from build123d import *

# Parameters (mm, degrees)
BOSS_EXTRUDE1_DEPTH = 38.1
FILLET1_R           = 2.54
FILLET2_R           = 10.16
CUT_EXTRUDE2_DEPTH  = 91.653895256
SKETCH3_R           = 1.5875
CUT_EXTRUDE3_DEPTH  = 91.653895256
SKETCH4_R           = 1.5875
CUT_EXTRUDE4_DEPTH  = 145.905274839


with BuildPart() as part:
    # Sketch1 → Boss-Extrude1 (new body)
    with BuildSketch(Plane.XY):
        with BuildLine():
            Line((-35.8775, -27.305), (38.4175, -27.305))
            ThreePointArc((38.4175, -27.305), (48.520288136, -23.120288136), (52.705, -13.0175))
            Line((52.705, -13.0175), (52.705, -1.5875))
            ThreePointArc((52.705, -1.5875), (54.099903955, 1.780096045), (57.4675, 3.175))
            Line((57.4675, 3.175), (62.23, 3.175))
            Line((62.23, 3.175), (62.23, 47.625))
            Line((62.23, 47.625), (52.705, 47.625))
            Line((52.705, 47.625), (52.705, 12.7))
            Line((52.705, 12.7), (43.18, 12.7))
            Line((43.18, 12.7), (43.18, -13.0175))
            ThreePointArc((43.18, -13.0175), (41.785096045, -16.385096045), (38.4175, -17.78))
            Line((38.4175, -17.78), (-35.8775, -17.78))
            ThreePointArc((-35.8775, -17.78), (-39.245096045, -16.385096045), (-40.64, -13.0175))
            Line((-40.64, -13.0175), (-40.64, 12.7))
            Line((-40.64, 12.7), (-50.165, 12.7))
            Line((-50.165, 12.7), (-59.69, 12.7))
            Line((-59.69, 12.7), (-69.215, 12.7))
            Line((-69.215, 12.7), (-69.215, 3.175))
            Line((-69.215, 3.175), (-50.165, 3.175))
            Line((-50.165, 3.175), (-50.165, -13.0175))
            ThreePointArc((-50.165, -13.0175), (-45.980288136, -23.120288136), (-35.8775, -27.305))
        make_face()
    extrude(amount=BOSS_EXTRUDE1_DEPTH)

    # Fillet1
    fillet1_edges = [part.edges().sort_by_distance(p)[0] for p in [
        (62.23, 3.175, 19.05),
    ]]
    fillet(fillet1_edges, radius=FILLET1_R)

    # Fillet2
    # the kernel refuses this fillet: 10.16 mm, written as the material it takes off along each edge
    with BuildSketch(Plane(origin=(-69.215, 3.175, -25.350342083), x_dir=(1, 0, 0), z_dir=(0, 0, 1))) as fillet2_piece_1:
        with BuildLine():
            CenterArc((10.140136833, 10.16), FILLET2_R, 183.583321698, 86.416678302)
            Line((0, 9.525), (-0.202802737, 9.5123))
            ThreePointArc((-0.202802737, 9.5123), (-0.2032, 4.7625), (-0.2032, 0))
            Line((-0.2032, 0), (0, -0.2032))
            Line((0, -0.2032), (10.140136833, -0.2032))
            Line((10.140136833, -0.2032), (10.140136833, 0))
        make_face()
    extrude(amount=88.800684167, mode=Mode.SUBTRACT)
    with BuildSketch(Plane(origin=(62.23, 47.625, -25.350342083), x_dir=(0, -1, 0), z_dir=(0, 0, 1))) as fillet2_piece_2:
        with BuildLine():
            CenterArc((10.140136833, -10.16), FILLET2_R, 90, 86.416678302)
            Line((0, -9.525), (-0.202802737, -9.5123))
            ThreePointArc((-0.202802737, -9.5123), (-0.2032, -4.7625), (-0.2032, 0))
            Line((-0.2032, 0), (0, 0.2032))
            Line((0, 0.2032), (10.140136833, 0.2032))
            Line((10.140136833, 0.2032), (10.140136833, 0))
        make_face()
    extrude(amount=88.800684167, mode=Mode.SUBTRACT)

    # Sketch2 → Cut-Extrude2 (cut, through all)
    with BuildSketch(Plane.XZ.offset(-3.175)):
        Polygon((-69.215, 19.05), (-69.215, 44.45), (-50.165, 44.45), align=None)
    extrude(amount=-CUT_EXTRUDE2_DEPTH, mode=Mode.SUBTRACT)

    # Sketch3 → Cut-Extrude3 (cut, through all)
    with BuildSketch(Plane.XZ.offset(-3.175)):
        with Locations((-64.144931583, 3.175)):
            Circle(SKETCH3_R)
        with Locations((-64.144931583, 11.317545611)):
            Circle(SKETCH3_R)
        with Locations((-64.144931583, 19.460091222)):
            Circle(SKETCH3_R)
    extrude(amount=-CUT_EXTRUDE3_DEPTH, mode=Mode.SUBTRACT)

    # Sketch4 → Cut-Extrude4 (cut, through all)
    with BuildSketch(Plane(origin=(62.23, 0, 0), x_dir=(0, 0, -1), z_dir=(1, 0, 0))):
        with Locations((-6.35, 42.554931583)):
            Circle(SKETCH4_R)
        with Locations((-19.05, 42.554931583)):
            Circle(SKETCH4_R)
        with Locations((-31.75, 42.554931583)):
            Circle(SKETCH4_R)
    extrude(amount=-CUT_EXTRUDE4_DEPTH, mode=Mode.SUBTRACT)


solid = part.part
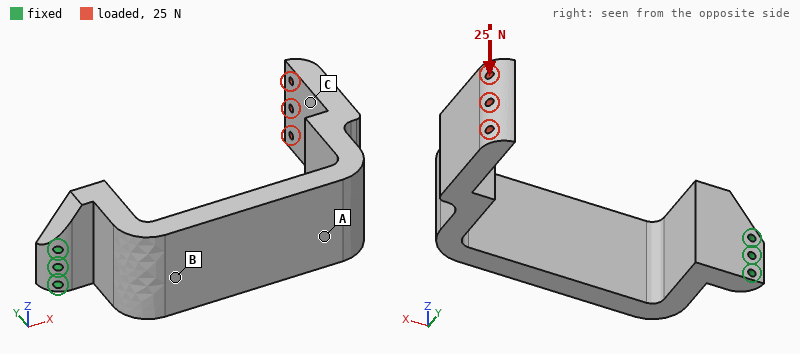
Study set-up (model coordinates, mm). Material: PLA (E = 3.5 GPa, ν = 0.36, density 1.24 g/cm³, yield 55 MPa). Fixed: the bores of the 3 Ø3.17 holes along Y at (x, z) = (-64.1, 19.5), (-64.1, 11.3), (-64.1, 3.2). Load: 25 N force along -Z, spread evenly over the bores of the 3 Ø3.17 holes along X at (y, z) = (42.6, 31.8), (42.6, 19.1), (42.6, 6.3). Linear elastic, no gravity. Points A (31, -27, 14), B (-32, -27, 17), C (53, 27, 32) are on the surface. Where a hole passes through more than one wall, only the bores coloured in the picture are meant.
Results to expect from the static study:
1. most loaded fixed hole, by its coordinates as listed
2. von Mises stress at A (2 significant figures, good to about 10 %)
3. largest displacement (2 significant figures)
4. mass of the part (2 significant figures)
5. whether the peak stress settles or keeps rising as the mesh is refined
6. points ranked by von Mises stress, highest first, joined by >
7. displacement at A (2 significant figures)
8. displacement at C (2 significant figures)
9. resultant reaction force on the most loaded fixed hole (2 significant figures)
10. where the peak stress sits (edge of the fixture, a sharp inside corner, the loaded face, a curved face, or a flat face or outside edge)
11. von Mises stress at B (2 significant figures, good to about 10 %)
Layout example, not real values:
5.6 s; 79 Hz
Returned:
(-64.1, 19.5); 2.4 MPa; 1.7 mm; 95 g; keeps rising; B > A > C; 0.41 mm; 1.4 mm; 180 N; edge of the fixture; 3.2 MPa
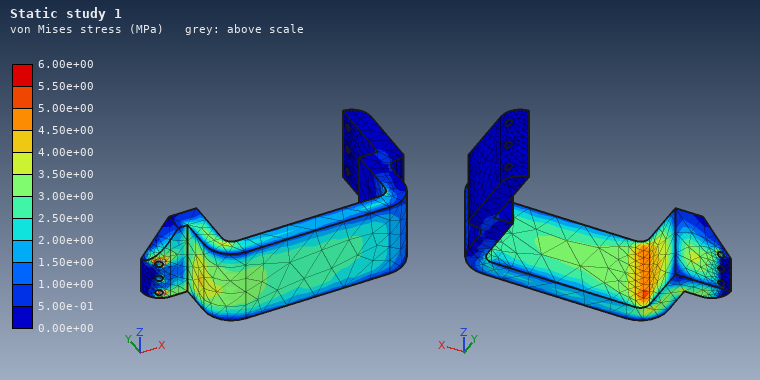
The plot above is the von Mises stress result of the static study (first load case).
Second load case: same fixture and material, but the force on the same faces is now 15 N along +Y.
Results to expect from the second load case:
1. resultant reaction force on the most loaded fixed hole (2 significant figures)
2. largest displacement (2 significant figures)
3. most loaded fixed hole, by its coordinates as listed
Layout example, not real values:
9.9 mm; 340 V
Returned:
20 N; 1.7 mm; (-64.1, 11.3)
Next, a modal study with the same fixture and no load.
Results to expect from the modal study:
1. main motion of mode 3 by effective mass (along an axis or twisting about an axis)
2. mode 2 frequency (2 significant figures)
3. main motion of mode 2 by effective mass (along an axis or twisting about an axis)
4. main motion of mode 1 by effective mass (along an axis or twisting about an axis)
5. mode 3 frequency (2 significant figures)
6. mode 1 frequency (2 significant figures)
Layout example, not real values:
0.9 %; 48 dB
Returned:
along X; 130 Hz; along Z; along Y; 270 Hz; 78 Hz
